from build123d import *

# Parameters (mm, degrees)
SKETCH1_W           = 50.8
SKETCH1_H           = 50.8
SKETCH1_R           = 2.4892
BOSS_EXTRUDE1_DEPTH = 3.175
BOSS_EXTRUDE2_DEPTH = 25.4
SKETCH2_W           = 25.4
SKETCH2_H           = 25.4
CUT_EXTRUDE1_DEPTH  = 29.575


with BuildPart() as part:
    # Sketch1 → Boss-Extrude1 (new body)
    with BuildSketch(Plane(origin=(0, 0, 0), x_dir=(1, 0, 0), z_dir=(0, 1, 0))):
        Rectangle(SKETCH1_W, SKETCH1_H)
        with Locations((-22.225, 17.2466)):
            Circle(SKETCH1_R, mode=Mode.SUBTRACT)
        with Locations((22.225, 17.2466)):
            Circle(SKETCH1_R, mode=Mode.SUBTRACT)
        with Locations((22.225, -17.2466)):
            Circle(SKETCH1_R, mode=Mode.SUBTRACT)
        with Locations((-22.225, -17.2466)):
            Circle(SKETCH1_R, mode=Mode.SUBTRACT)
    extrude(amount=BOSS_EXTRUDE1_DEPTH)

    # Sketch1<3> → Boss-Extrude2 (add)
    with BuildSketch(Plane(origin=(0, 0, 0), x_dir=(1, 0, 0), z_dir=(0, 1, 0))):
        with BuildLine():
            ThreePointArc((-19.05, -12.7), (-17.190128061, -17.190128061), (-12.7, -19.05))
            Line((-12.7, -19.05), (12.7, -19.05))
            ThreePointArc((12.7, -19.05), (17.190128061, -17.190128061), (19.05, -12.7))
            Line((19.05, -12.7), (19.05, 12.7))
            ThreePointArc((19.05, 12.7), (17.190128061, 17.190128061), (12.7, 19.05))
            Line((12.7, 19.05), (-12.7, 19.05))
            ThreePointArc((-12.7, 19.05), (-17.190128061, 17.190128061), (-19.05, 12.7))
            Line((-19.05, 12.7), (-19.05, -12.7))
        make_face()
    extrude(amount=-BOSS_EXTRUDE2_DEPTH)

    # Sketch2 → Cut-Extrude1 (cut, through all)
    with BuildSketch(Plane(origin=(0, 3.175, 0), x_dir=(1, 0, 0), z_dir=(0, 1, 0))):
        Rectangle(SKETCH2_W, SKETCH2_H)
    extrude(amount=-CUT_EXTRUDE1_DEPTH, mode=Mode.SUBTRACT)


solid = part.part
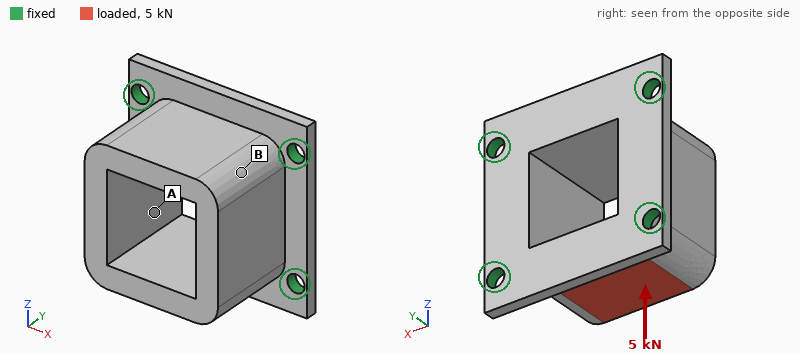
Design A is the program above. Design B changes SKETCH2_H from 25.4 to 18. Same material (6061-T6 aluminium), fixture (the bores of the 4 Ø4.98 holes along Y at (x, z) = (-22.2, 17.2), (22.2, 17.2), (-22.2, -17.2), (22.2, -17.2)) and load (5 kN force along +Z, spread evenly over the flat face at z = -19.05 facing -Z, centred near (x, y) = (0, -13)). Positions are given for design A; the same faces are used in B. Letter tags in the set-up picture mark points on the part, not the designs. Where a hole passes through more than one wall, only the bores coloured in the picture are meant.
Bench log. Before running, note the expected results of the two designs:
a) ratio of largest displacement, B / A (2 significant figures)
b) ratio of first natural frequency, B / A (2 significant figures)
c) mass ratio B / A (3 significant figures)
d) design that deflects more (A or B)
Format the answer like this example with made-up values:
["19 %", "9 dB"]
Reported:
["0.69", "0.93", "1.21", "A"]
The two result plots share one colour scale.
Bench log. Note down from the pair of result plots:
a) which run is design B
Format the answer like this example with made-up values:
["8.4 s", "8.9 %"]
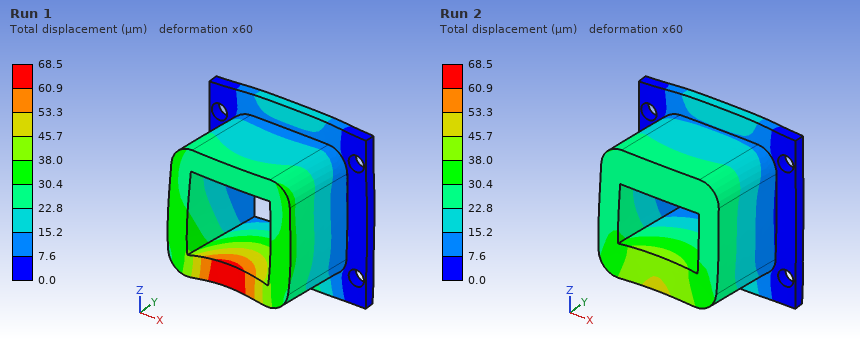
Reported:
["Run 2"]
